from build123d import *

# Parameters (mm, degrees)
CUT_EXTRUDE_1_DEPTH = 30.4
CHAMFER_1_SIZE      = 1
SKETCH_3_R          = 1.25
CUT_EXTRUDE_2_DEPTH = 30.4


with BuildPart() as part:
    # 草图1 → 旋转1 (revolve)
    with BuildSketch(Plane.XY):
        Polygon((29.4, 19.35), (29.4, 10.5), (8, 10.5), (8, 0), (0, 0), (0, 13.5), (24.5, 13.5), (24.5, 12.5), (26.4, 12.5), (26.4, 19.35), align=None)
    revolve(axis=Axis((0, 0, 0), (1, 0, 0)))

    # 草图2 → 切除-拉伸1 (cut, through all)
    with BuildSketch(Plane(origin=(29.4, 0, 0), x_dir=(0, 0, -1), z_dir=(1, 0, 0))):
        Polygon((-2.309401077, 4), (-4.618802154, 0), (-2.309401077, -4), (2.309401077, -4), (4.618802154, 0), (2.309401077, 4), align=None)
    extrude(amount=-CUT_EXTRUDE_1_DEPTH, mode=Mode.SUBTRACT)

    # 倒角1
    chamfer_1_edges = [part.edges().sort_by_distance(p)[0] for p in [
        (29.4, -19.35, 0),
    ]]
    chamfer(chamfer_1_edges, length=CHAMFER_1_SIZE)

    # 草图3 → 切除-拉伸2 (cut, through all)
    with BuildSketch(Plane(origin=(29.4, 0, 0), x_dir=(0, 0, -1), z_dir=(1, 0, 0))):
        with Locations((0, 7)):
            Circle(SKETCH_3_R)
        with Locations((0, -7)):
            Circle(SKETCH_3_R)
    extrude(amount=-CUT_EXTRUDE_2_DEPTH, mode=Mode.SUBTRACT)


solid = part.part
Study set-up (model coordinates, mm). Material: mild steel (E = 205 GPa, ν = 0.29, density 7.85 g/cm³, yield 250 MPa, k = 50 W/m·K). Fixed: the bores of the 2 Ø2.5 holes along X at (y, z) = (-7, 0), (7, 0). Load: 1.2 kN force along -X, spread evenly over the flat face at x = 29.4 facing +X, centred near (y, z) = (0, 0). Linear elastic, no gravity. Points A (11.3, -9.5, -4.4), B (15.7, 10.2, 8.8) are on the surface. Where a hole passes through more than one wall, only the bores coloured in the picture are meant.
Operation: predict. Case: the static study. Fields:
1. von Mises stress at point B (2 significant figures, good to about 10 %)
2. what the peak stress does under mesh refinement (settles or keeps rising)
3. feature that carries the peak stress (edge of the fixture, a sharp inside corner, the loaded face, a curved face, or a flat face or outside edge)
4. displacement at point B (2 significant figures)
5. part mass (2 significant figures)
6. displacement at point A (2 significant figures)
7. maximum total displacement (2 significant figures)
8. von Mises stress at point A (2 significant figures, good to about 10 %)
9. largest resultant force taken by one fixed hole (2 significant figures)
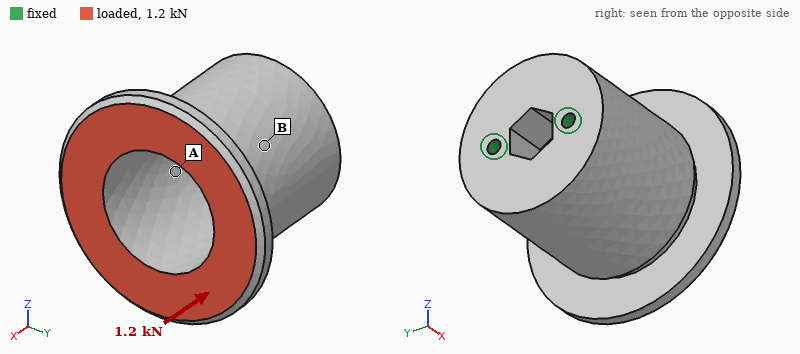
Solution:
4.9 MPa
keeps rising
edge of the fixture
0.86 µm
82 g
0.72 µm
4.8 µm
10 MPa
600 N
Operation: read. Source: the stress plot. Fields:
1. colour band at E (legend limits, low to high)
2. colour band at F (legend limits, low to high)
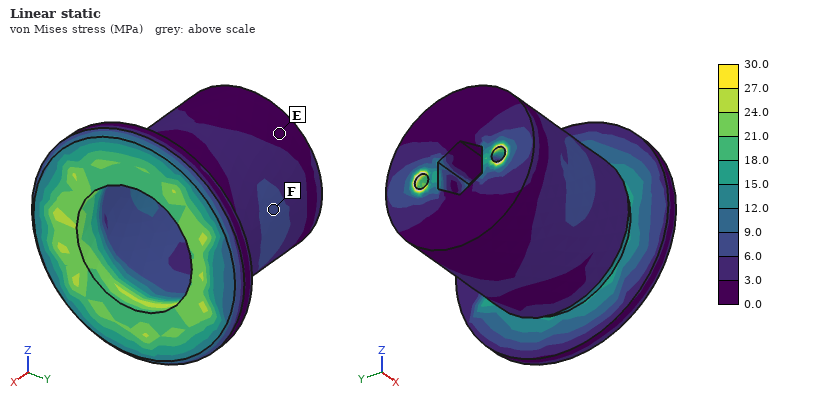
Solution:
0.0 to 3.0 MPa
6.0 to 9.0 MPa
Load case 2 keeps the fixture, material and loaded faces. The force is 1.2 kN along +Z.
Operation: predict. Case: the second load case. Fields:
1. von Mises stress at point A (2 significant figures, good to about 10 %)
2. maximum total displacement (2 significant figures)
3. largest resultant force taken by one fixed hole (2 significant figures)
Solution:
23 MPa
24 µm
600 N
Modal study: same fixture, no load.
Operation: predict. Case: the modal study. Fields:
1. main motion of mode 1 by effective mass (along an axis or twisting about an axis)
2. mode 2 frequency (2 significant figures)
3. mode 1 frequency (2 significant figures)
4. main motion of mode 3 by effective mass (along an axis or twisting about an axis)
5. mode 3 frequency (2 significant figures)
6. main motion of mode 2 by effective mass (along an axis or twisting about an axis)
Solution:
along Z
11 kHz
7000 Hz
twisting about X
16 kHz
along Y
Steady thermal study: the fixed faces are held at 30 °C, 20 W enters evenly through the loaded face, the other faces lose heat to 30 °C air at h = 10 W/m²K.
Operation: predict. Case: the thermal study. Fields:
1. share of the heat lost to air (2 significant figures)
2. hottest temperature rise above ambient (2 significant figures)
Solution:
7.6 %
51 K
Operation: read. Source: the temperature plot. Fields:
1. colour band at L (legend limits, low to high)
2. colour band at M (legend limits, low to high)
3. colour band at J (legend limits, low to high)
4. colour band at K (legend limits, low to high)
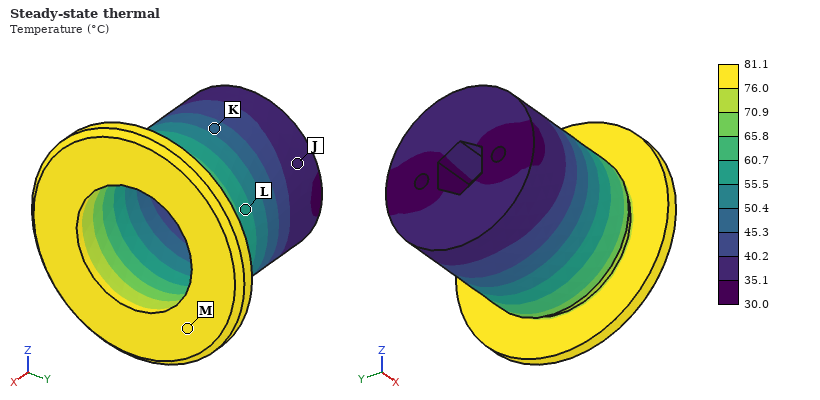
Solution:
55.5 to 60.7 °C
76.0 to 81.1 °C
35.1 to 40.2 °C
45.3 to 50.4 °C
